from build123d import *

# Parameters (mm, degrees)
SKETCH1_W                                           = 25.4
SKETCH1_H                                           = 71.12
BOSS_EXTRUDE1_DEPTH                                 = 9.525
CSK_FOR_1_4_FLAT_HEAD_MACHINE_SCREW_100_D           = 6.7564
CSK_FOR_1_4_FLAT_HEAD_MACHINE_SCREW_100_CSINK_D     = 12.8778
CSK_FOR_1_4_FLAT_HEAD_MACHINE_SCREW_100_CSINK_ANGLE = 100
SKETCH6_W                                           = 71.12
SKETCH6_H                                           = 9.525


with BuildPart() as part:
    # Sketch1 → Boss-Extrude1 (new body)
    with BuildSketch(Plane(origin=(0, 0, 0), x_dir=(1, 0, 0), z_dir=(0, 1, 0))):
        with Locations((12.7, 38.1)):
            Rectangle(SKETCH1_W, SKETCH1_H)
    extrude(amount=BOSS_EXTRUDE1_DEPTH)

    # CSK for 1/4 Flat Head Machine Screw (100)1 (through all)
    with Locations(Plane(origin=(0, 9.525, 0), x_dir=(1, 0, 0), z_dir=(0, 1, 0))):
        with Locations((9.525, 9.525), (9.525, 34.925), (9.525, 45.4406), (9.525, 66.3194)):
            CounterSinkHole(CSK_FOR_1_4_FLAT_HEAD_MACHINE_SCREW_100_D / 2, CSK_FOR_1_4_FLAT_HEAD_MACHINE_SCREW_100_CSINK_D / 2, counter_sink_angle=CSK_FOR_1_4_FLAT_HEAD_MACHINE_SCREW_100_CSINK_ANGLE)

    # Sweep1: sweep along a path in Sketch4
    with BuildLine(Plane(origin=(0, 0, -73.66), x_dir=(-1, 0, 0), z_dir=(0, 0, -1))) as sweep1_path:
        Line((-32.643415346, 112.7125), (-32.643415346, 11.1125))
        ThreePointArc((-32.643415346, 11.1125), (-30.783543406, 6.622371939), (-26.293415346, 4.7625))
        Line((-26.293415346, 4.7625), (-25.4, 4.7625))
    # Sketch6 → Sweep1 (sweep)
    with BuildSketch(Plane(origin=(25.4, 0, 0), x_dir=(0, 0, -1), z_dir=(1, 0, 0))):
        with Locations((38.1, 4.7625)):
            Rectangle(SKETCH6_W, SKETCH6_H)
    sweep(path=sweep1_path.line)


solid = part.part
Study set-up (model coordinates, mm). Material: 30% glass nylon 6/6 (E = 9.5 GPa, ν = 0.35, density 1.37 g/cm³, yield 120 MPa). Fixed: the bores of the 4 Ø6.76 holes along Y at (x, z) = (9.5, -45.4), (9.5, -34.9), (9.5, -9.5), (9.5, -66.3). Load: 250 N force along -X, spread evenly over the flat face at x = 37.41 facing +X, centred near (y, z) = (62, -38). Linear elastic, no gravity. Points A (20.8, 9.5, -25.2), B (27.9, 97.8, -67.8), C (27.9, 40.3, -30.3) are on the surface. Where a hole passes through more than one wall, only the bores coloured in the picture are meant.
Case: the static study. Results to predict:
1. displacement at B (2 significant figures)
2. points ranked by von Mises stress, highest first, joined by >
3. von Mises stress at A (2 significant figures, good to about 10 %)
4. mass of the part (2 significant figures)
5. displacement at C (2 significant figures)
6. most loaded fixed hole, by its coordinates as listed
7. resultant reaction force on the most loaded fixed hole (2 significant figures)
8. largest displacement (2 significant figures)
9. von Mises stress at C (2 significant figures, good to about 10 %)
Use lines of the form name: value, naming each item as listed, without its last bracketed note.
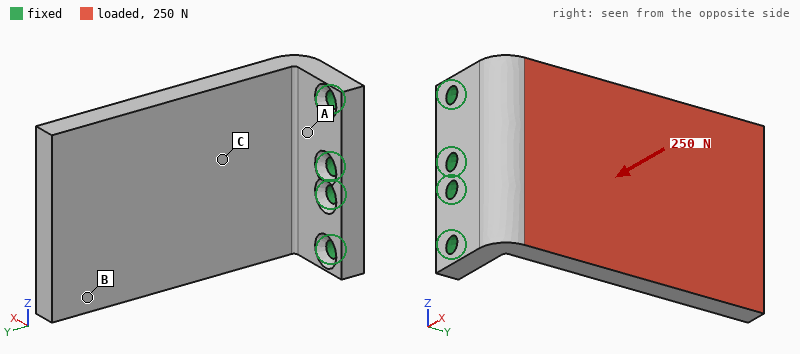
displacement at B: 1.2 mm
points ranked by von Mises stress, highest first, joined by >: A > C > B
von Mises stress at A: 12 MPa
mass of the part: 130 g
displacement at C: 0.36 mm
most loaded fixed hole, by its coordinates as listed: (9.5, -34.9)
resultant reaction force on the most loaded fixed hole: 110 N
largest displacement: 1.5 mm
von Mises stress at C: 5.6 MPa
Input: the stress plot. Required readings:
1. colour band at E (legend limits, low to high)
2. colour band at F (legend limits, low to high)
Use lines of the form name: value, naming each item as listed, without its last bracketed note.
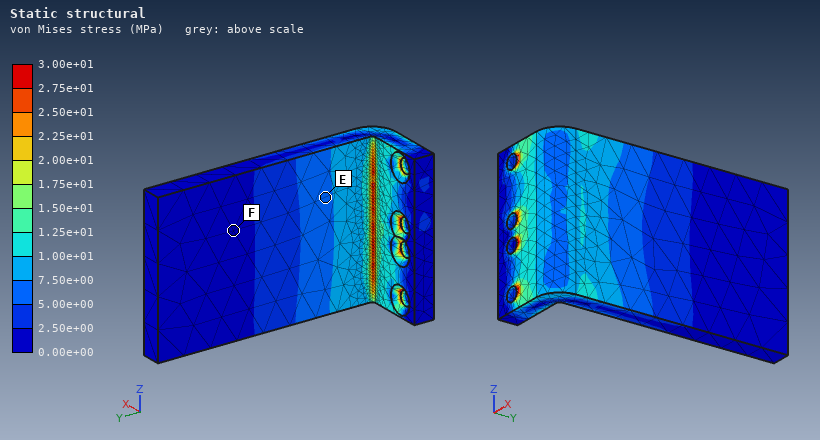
colour band at E: 5.00e+00 to 7.50e+00 MPa
colour band at F: 0.00e+00 to 2.50e+00 MPa
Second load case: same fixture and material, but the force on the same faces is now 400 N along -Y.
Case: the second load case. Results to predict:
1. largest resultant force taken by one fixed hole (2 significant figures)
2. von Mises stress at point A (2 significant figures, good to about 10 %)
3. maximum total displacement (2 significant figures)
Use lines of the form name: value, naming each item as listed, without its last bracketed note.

largest resultant force taken by one fixed hole: 110 N
von Mises stress at point A: 5.4 MPa
maximum total displacement: 0.52 mm
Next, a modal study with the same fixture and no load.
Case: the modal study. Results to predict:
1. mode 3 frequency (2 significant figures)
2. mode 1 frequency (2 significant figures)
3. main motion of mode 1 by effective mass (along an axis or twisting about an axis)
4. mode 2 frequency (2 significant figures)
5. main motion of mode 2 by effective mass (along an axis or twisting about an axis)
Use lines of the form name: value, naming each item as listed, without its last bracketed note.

mode 3 frequency: 1100 Hz
mode 1 frequency: 260 Hz
main motion of mode 1 by effective mass: along X
mode 2 frequency: 700 Hz
main motion of mode 2 by effective mass: along Z
